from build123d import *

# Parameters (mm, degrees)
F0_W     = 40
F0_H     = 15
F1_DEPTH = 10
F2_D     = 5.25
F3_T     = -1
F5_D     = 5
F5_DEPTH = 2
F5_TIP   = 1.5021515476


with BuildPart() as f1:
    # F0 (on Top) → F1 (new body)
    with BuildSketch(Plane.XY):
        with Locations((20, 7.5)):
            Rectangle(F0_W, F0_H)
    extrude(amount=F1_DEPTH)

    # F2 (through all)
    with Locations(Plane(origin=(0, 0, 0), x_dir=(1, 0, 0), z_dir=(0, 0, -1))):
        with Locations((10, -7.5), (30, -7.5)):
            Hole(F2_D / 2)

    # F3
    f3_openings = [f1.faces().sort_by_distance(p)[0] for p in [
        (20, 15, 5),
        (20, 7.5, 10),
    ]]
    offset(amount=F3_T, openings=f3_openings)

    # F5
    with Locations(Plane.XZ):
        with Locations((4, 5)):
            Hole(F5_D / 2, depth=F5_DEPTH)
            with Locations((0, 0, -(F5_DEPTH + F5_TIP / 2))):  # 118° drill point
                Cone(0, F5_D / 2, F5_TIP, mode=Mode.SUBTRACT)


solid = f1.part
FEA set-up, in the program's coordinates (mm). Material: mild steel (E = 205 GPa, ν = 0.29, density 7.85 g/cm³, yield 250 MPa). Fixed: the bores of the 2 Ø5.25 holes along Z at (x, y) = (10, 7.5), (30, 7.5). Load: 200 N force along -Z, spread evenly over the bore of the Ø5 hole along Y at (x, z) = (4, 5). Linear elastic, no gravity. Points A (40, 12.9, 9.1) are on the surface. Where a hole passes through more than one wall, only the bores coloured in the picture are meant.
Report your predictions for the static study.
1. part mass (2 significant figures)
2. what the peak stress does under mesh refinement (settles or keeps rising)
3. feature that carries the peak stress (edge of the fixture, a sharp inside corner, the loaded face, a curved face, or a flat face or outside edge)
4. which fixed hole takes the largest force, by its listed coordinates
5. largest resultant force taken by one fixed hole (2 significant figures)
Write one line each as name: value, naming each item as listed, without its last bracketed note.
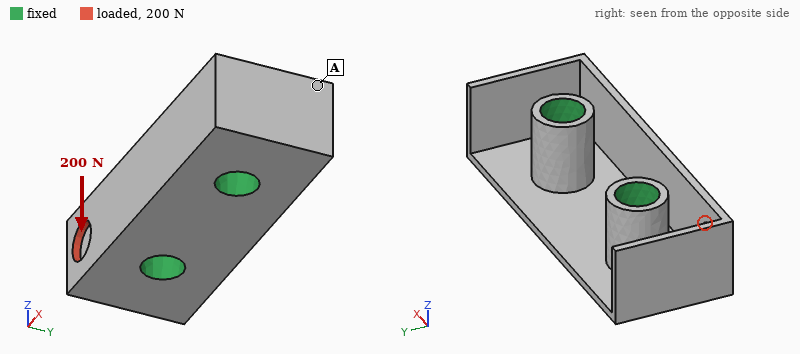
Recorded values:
part mass: 12 g
what the peak stress does under mesh refinement: keeps rising
feature that carries the peak stress: edge of the fixture
which fixed hole takes the largest force, by its listed coordinates: (10, 7.5)
largest resultant force taken by one fixed hole: 240 N
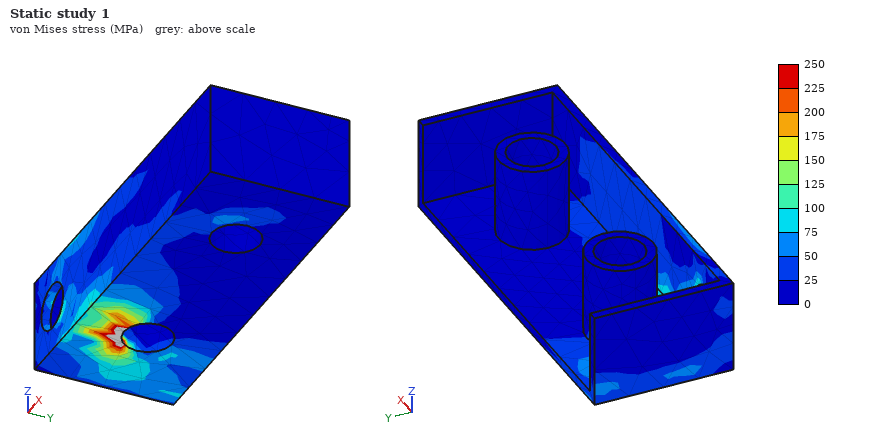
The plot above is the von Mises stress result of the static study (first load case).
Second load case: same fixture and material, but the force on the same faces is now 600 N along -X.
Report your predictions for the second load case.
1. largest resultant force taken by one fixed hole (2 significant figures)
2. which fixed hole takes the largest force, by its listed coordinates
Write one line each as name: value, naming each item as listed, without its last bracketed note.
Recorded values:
largest resultant force taken by one fixed hole: 400 N
which fixed hole takes the largest force, by its listed coordinates: (10, 7.5)
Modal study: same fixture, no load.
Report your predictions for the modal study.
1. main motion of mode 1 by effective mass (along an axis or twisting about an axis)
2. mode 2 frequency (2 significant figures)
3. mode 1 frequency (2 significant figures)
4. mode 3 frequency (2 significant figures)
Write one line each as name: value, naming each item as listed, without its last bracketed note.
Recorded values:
main motion of mode 1 by effective mass: along Y
mode 2 frequency: 6300 Hz
mode 1 frequency: 5500 Hz
mode 3 frequency: 7900 Hz
